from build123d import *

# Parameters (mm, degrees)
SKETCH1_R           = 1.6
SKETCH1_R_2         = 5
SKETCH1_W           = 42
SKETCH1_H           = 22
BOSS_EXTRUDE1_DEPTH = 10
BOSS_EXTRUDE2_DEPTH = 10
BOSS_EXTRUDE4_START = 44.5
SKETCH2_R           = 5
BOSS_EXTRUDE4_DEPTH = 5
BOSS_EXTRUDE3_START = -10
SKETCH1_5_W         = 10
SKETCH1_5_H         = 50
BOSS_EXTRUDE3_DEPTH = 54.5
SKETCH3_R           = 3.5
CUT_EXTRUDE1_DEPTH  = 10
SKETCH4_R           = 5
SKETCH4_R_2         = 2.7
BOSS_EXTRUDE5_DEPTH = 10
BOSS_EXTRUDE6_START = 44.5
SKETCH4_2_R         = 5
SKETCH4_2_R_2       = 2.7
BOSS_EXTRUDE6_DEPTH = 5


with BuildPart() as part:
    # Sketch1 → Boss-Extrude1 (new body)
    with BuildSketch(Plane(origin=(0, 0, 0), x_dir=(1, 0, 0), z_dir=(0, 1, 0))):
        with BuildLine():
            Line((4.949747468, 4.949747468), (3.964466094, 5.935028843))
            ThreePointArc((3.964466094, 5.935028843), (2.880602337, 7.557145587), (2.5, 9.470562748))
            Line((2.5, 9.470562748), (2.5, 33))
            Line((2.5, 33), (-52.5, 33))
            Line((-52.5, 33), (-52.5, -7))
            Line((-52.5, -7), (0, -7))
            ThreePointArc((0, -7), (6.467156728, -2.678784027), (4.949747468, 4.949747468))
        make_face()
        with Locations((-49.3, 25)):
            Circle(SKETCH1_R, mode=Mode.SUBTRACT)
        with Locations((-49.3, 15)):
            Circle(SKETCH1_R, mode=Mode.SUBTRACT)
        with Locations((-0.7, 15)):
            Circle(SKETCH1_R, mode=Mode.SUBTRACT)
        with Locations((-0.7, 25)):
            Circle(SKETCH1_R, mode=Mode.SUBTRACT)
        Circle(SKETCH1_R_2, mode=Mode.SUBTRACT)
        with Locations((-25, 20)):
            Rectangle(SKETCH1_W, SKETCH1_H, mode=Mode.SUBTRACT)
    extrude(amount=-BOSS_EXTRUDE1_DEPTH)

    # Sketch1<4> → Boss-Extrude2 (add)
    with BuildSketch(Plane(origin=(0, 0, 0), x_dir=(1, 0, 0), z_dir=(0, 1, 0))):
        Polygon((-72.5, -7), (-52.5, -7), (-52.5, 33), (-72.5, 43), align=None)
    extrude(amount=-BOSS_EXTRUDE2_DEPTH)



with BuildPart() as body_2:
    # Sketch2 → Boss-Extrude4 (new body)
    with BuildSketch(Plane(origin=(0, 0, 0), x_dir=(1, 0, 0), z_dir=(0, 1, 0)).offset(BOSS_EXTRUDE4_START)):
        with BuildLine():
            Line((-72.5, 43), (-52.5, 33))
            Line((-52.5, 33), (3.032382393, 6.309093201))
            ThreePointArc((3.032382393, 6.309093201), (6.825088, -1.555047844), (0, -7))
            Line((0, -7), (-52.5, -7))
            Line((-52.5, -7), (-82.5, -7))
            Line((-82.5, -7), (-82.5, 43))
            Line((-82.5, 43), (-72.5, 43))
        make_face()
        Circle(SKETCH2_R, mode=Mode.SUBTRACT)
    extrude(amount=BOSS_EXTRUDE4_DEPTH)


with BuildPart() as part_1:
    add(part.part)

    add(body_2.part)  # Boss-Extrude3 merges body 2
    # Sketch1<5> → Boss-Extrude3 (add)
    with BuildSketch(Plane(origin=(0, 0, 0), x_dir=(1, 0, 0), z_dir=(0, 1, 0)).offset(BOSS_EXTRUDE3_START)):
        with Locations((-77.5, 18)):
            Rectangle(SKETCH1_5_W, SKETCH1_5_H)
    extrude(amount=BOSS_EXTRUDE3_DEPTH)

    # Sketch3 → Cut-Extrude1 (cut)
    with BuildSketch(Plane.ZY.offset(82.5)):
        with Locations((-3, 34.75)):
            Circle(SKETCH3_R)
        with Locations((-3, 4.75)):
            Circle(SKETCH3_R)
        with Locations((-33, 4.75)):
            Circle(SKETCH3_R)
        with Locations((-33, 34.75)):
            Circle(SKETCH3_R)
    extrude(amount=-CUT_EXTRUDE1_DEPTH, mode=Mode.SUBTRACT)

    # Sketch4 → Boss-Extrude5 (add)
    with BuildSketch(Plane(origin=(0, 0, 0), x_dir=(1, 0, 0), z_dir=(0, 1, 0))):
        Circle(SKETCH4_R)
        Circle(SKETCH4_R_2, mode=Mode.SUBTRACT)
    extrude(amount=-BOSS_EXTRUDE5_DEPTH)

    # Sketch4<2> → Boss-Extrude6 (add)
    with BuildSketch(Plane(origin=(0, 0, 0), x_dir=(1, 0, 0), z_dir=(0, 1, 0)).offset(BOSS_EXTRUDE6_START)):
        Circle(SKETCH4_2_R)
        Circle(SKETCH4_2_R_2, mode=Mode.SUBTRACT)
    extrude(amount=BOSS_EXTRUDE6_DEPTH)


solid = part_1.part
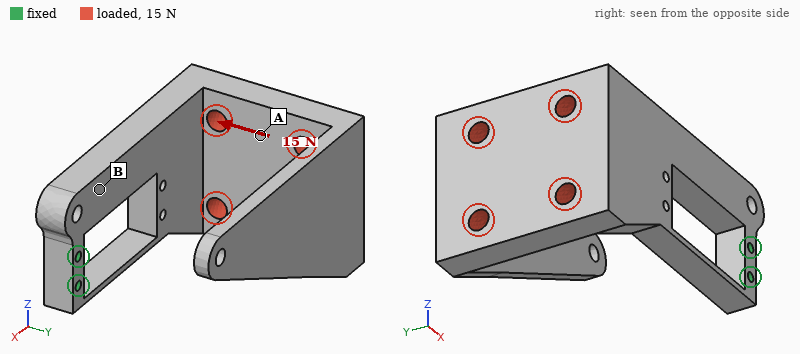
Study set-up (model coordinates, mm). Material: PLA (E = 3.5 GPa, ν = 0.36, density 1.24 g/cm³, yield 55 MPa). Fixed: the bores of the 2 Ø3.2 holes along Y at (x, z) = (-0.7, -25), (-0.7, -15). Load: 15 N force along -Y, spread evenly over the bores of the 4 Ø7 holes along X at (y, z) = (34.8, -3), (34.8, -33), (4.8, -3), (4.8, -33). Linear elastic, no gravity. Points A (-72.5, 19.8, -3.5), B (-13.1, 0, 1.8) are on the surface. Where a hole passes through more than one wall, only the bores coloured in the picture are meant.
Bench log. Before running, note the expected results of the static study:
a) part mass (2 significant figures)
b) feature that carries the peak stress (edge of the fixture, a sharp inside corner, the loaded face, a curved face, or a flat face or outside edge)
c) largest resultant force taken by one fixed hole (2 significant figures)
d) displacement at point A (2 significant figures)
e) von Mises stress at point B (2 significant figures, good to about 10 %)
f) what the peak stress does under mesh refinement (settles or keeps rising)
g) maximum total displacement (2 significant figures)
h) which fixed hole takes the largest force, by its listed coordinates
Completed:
77 g
edge of the fixture
8.1 N
0.93 mm
2.5 MPa
keeps rising
1.3 mm
(-0.7, -15)
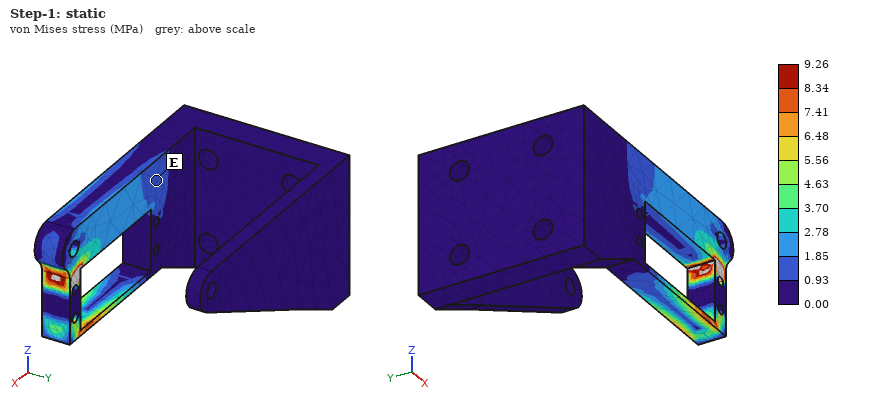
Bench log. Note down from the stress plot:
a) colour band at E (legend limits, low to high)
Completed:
0.93 to 1.85 MPa
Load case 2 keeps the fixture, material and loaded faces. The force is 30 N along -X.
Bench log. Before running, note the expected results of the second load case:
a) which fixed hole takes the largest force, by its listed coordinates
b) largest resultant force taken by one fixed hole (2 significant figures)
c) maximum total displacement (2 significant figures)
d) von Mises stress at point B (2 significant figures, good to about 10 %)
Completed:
(-0.7, -15)
19 N
1.1 mm
2.1 MPa
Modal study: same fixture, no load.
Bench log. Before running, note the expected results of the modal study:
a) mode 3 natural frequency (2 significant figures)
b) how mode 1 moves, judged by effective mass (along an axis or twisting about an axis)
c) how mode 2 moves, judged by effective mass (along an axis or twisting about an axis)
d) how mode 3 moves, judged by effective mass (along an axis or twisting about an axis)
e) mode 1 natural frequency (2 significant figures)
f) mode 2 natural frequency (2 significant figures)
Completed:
220 Hz
along Y
along Z
along Y
78 Hz
120 Hz
